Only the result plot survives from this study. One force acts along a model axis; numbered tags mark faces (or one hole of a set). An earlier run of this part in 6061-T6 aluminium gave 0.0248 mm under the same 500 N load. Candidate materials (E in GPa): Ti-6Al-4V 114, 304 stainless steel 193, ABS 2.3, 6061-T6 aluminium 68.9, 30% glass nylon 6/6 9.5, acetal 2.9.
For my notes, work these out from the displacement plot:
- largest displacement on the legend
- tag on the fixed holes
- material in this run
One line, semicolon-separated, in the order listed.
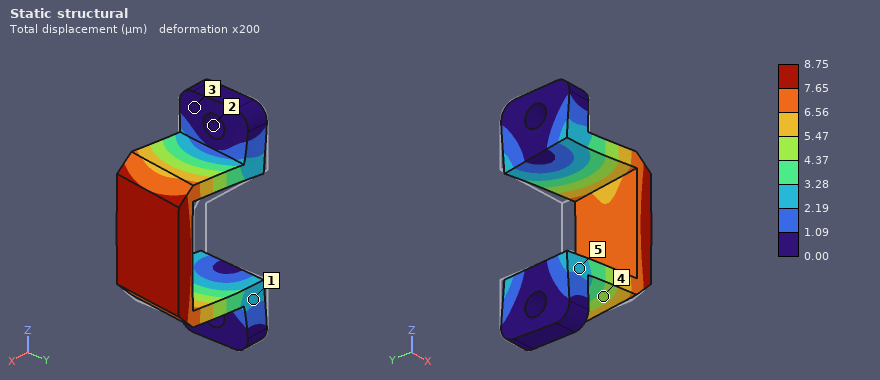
8.75 µm; 2; 304 stainless steel
